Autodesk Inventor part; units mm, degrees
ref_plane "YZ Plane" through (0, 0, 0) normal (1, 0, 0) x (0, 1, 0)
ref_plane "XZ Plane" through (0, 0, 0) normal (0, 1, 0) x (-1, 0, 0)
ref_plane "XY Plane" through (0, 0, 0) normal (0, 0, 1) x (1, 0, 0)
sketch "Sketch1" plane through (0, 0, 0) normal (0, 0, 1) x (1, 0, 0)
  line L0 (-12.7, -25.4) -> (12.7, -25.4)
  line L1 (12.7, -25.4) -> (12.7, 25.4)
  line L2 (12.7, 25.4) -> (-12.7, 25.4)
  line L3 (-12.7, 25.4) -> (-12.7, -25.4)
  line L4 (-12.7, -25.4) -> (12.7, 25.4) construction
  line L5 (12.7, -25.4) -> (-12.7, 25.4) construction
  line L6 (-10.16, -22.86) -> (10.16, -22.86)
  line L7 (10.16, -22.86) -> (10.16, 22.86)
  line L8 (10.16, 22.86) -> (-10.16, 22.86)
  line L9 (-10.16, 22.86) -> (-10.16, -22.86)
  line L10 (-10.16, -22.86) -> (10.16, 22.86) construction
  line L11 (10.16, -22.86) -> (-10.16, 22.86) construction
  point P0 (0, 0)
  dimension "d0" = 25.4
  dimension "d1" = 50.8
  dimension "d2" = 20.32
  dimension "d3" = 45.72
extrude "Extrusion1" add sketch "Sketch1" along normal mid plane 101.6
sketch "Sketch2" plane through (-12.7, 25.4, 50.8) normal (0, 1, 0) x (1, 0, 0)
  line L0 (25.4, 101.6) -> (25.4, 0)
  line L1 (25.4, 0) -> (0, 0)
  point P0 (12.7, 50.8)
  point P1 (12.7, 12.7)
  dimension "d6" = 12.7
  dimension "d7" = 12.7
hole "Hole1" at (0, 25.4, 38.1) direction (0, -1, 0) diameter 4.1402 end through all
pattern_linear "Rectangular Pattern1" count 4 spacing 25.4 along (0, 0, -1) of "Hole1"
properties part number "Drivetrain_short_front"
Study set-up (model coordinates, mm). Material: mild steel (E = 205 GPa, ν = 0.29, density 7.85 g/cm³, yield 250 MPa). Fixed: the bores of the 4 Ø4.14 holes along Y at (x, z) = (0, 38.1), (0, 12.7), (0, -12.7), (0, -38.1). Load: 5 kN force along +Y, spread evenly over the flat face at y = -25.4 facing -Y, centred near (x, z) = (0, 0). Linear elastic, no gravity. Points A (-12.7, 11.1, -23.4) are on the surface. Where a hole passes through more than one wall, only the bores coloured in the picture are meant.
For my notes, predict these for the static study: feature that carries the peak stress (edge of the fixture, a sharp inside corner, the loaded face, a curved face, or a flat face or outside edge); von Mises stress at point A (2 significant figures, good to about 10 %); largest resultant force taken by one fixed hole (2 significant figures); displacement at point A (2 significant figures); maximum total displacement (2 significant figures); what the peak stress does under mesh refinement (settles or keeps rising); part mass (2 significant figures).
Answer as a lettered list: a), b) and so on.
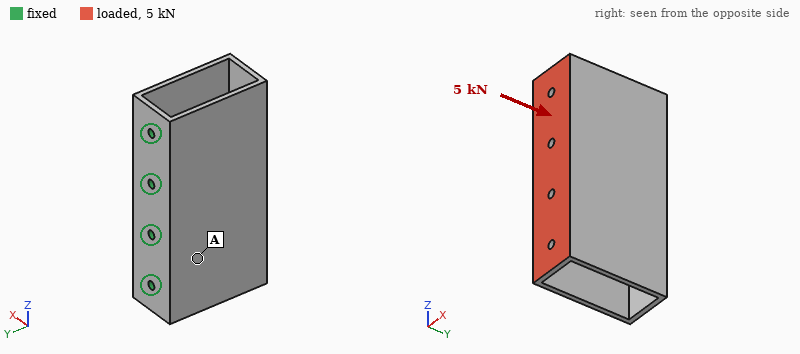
a) edge of the fixture
b) 26 MPa
c) 1.3 kN
d) 41 µm
e) 52 µm
f) keeps rising
g) 290 g
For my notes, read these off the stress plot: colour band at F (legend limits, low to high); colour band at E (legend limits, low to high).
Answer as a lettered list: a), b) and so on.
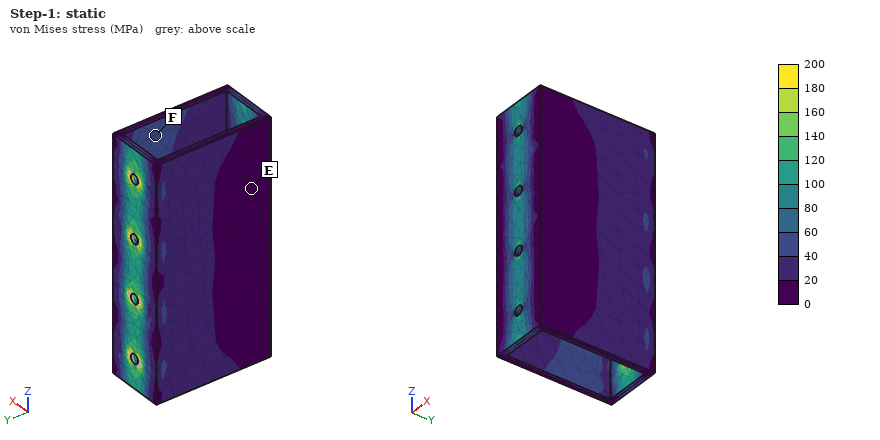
a) 40 to 60 MPa
b) 0 to 20 MPa
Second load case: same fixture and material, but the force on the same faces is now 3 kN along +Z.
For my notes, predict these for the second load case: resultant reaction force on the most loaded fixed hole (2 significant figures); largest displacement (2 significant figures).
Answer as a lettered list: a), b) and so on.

a) 1.8 kN
b) 72 µm
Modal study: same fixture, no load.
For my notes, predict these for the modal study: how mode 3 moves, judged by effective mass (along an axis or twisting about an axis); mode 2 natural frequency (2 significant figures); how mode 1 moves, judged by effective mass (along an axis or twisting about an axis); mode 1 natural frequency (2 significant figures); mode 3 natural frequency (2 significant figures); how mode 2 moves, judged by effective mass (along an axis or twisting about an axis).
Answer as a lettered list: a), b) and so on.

a) along Z
b) 2200 Hz
c) along X
d) 670 Hz
e) 2800 Hz
f) twisting about Y
